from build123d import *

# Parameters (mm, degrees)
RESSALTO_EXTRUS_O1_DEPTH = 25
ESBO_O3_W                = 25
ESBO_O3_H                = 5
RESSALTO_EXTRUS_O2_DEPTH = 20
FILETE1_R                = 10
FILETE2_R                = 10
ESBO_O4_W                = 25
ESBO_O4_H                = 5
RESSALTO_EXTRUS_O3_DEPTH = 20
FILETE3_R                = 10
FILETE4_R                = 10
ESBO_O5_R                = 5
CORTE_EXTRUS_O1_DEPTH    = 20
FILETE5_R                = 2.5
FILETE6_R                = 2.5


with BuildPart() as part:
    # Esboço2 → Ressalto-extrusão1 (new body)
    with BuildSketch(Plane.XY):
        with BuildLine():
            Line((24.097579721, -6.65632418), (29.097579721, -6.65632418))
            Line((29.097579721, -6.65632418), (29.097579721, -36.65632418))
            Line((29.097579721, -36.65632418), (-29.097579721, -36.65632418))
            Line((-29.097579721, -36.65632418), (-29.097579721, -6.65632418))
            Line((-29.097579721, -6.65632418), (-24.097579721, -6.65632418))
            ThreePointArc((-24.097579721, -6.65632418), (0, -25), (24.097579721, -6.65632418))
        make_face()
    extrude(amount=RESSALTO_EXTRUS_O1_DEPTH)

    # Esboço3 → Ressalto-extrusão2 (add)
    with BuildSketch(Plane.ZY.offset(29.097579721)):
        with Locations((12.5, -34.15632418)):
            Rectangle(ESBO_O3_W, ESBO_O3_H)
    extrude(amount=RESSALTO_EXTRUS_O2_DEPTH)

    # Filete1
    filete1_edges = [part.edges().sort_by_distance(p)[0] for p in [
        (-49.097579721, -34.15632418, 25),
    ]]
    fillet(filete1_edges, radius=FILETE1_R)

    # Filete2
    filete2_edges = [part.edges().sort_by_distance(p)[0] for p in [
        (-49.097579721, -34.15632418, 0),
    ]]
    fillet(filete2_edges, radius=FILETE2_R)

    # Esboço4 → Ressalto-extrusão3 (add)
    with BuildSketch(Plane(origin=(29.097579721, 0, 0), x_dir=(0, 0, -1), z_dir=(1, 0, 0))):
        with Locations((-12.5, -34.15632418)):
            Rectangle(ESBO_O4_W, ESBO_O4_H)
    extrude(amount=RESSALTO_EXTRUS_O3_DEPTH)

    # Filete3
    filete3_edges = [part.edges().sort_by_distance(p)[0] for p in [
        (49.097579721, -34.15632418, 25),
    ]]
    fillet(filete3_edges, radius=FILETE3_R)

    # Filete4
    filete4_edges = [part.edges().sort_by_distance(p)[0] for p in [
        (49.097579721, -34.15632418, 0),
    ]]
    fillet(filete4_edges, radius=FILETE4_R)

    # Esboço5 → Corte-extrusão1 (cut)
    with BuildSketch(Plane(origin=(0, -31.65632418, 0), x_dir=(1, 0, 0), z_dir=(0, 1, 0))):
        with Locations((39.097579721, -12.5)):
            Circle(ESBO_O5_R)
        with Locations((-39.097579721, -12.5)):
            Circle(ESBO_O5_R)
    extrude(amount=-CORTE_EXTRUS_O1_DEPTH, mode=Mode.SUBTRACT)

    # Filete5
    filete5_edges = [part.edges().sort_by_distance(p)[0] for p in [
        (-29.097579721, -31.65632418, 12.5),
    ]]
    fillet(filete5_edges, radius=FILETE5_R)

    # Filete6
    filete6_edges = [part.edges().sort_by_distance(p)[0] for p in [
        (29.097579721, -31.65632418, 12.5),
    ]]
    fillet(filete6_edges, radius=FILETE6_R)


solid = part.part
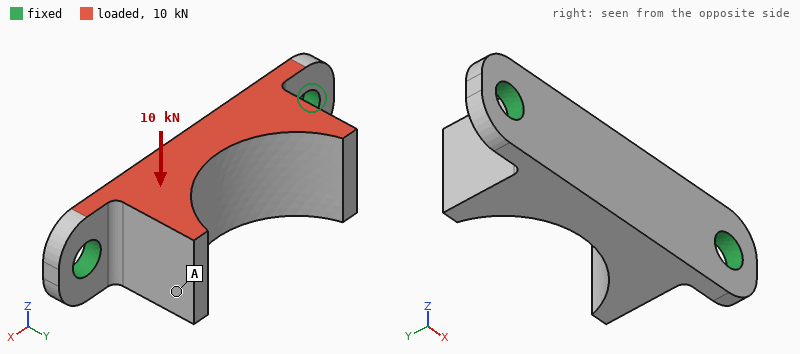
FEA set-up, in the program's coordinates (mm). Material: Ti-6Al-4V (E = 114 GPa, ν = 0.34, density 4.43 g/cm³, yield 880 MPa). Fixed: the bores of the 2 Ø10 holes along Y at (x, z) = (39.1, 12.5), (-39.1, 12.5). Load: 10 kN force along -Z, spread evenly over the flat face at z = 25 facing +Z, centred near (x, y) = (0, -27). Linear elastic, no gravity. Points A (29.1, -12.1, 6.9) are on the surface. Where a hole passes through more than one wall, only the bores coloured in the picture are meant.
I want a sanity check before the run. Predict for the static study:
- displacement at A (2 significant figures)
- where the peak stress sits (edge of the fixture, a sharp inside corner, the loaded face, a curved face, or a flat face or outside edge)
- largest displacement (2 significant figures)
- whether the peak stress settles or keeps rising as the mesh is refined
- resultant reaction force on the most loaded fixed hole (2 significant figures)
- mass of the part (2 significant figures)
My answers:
0.11 mm
edge of the fixture
0.14 mm
keeps rising
5.0 kN
140 g
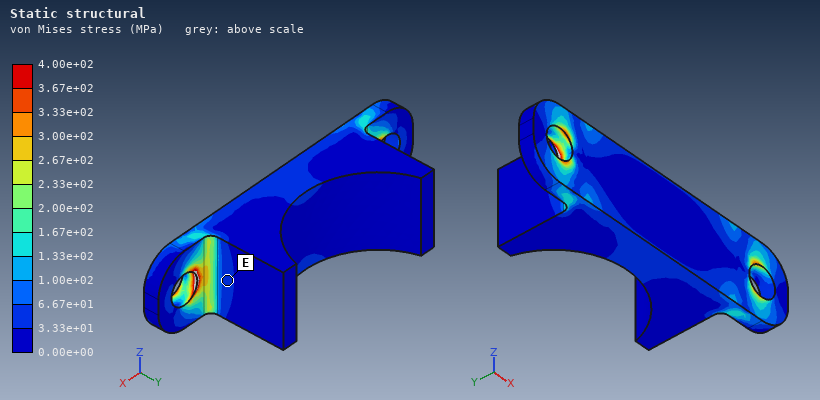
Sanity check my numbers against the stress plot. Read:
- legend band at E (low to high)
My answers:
3.33e+01 to 6.67e+01 MPa
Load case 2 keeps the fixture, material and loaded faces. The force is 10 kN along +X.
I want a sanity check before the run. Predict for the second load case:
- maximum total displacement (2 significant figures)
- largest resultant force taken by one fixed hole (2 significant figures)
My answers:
24 µm
5.4 kN
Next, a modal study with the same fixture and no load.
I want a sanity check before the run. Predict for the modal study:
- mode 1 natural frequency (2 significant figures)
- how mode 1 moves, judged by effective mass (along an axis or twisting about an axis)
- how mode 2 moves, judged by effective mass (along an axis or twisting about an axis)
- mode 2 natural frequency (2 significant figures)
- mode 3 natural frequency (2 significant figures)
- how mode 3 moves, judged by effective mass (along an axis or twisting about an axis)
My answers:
4500 Hz
along Z
along Y
6400 Hz
10 kHz
twisting about Y
